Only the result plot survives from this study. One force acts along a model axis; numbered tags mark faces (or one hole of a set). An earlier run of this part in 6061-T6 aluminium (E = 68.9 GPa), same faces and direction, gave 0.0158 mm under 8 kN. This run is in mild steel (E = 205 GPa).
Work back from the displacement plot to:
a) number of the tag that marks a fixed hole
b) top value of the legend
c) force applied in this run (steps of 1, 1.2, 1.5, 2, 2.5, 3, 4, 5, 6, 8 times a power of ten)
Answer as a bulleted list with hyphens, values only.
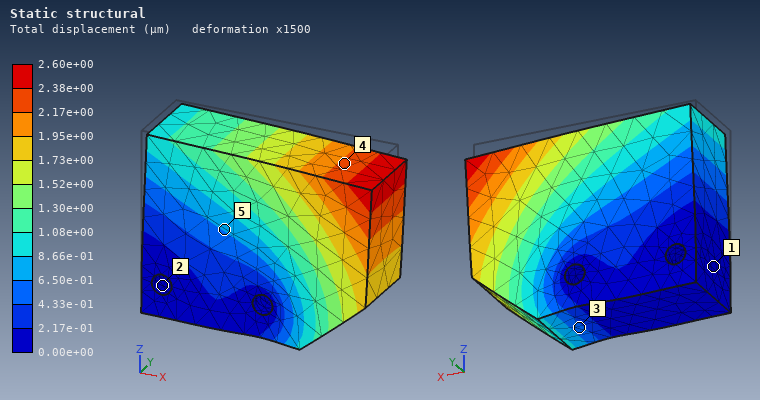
- 2
- 2.60e+00 µm
- 4 kN
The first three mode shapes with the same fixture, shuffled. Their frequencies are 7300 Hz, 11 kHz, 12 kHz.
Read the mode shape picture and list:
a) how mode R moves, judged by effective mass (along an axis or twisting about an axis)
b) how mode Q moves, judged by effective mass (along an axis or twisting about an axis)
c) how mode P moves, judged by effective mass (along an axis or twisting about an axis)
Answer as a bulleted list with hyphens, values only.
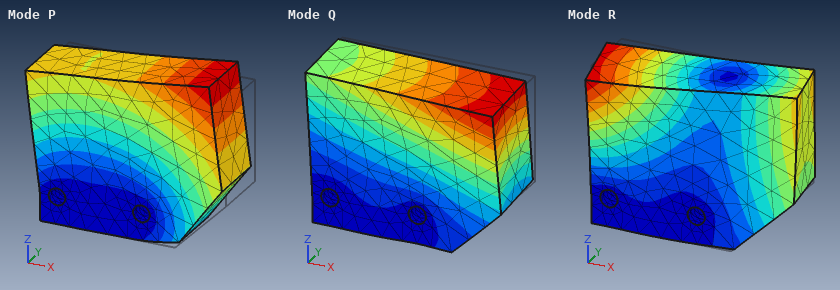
- twisting about Z
- along Y
- along X
